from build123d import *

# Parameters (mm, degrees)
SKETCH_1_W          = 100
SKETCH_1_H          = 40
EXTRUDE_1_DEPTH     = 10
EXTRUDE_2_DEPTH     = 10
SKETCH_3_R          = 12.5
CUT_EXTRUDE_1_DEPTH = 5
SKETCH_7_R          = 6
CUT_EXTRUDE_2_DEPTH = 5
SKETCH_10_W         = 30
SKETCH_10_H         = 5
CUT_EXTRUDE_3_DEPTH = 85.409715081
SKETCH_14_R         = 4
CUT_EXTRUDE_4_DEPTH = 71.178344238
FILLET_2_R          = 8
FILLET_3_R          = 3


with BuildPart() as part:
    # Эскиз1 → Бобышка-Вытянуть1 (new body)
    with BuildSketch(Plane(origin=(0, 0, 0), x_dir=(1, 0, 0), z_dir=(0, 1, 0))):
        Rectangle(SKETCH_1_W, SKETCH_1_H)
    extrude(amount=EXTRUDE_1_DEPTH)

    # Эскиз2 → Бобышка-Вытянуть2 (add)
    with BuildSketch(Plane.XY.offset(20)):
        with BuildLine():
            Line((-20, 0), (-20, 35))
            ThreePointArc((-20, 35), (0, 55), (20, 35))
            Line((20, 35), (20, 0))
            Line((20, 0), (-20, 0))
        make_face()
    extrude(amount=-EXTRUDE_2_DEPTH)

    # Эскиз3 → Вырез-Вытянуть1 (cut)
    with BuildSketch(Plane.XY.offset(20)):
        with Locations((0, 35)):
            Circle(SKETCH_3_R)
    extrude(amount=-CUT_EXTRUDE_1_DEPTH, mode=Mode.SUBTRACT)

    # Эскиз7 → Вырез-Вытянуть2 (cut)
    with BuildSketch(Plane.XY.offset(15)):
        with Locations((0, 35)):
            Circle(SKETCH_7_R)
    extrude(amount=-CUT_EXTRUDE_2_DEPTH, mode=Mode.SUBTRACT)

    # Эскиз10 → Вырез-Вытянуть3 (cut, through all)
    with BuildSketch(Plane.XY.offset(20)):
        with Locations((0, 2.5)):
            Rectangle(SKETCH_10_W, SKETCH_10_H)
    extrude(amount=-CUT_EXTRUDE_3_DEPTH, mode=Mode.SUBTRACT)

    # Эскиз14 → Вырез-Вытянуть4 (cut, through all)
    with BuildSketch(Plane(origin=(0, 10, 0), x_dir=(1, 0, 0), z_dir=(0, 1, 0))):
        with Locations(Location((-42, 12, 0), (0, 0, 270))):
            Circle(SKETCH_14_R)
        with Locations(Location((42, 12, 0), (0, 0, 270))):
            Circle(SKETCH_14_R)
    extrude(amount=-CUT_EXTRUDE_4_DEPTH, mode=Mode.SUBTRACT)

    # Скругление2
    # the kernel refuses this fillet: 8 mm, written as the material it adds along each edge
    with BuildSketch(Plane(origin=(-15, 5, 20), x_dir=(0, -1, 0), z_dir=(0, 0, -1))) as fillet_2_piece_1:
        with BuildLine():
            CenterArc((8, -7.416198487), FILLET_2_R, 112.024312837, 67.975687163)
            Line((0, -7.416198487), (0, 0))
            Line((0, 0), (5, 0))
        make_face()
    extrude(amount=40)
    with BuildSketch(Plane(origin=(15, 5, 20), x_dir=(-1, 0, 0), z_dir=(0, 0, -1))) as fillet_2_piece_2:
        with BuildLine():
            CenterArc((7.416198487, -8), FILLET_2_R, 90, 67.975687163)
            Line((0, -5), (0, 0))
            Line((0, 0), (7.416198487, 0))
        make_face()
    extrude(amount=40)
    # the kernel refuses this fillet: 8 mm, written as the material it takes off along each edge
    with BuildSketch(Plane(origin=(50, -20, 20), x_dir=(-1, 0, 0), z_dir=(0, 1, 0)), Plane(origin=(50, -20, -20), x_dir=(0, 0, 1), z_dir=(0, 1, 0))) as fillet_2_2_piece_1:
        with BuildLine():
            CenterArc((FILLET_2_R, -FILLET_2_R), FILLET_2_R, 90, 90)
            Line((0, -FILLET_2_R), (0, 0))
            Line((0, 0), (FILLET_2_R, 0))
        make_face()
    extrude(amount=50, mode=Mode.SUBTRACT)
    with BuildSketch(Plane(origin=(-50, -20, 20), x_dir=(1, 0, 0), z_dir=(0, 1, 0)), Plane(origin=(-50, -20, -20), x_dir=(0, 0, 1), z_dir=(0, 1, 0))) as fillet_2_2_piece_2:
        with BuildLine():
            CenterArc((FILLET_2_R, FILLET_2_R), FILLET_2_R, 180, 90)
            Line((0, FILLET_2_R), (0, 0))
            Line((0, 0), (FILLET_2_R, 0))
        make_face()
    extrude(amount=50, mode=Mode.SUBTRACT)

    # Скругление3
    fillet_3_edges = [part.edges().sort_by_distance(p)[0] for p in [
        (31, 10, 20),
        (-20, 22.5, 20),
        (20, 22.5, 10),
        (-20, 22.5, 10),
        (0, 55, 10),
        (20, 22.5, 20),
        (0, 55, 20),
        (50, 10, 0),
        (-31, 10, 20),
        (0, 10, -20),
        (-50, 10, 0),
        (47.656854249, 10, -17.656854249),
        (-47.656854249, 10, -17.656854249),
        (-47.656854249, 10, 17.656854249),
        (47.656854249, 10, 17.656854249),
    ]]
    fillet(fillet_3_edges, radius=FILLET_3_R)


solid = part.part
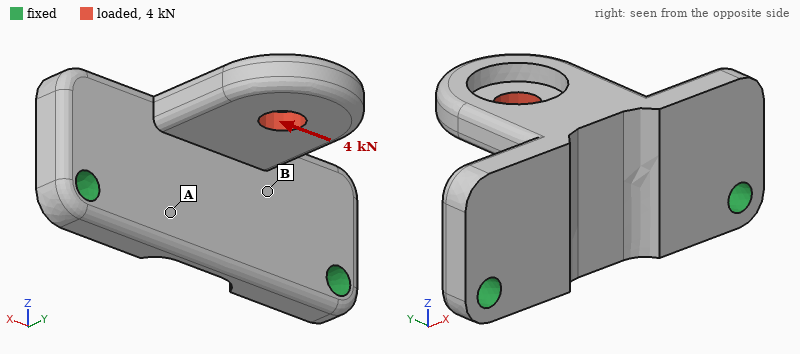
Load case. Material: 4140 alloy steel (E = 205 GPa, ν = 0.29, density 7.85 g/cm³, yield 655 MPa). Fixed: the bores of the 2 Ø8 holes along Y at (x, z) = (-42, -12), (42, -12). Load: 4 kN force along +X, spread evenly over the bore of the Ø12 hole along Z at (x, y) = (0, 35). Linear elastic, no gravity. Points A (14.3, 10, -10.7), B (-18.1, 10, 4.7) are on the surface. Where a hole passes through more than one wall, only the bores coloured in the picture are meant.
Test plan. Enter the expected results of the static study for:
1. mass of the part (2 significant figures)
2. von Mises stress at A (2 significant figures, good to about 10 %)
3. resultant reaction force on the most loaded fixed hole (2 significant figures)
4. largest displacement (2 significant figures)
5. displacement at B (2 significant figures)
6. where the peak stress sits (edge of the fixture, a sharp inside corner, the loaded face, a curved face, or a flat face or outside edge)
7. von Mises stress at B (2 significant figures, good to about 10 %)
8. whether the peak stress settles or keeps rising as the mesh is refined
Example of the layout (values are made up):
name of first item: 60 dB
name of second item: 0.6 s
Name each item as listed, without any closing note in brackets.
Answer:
mass of the part: 360 g
von Mises stress at A: 24 MPa
resultant reaction force on the most loaded fixed hole: 2.9 kN
largest displacement: 73 µm
displacement at B: 13 µm
where the peak stress sits: a sharp inside corner
von Mises stress at B: 55 MPa
whether the peak stress settles or keeps rising as the mesh is refined: keeps rising
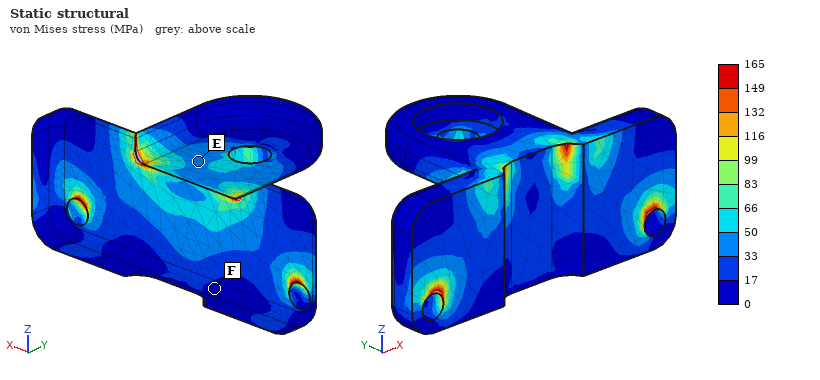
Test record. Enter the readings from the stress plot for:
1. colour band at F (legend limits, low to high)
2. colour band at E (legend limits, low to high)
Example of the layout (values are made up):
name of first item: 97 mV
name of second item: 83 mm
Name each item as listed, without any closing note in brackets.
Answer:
colour band at F: 0 to 17 MPa
colour band at E: 33 to 50 MPa
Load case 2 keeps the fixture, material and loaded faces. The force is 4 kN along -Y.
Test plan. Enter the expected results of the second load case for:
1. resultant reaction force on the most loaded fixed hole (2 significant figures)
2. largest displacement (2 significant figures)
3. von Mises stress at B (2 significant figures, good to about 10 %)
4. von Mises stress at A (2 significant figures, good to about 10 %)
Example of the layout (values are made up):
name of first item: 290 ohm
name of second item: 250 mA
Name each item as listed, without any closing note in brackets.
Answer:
resultant reaction force on the most loaded fixed hole: 2.2 kN
largest displacement: 82 µm
von Mises stress at B: 26 MPa
von Mises stress at A: 29 MPa
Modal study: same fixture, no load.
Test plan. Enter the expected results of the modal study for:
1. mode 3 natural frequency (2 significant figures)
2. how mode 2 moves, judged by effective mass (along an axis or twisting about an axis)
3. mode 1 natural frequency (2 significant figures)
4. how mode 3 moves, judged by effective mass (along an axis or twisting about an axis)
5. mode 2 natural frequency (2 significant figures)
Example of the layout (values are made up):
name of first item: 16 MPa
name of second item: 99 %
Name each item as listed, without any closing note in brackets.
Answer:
mode 3 natural frequency: 4500 Hz
how mode 2 moves, judged by effective mass: along Y
mode 1 natural frequency: 2200 Hz
how mode 3 moves, judged by effective mass: along X
mode 2 natural frequency: 4200 Hz
